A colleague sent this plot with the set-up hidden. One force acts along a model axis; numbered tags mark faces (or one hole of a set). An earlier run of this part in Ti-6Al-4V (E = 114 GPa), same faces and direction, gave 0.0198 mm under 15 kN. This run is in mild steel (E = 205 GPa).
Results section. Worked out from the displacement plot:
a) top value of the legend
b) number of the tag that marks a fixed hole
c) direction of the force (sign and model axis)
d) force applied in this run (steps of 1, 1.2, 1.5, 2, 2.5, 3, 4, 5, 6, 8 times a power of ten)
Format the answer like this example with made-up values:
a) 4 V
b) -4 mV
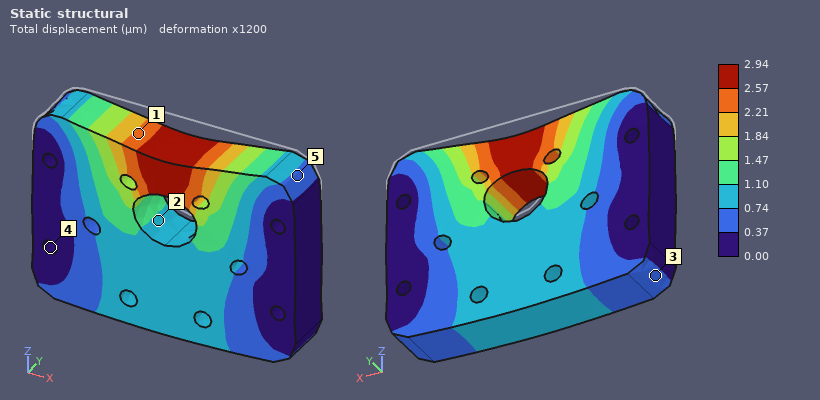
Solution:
a) 2.94 µm
b) 4
c) -Z
d) 4 kN
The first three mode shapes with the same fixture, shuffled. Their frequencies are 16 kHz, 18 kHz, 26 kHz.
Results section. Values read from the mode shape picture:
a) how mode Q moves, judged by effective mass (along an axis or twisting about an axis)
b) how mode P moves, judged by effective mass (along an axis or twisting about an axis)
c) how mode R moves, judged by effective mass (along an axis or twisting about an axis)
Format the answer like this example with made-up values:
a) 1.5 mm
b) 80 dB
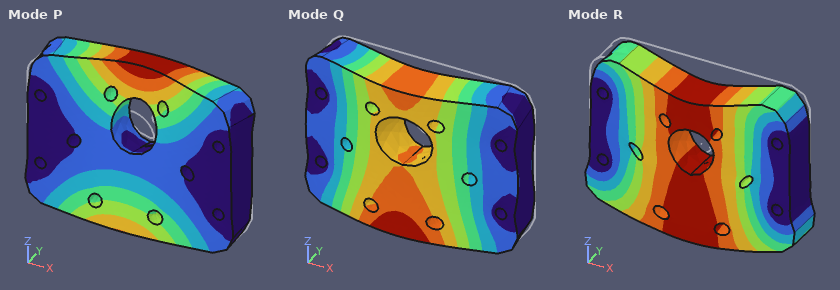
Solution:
a) along Y
b) twisting about X
c) along Z
